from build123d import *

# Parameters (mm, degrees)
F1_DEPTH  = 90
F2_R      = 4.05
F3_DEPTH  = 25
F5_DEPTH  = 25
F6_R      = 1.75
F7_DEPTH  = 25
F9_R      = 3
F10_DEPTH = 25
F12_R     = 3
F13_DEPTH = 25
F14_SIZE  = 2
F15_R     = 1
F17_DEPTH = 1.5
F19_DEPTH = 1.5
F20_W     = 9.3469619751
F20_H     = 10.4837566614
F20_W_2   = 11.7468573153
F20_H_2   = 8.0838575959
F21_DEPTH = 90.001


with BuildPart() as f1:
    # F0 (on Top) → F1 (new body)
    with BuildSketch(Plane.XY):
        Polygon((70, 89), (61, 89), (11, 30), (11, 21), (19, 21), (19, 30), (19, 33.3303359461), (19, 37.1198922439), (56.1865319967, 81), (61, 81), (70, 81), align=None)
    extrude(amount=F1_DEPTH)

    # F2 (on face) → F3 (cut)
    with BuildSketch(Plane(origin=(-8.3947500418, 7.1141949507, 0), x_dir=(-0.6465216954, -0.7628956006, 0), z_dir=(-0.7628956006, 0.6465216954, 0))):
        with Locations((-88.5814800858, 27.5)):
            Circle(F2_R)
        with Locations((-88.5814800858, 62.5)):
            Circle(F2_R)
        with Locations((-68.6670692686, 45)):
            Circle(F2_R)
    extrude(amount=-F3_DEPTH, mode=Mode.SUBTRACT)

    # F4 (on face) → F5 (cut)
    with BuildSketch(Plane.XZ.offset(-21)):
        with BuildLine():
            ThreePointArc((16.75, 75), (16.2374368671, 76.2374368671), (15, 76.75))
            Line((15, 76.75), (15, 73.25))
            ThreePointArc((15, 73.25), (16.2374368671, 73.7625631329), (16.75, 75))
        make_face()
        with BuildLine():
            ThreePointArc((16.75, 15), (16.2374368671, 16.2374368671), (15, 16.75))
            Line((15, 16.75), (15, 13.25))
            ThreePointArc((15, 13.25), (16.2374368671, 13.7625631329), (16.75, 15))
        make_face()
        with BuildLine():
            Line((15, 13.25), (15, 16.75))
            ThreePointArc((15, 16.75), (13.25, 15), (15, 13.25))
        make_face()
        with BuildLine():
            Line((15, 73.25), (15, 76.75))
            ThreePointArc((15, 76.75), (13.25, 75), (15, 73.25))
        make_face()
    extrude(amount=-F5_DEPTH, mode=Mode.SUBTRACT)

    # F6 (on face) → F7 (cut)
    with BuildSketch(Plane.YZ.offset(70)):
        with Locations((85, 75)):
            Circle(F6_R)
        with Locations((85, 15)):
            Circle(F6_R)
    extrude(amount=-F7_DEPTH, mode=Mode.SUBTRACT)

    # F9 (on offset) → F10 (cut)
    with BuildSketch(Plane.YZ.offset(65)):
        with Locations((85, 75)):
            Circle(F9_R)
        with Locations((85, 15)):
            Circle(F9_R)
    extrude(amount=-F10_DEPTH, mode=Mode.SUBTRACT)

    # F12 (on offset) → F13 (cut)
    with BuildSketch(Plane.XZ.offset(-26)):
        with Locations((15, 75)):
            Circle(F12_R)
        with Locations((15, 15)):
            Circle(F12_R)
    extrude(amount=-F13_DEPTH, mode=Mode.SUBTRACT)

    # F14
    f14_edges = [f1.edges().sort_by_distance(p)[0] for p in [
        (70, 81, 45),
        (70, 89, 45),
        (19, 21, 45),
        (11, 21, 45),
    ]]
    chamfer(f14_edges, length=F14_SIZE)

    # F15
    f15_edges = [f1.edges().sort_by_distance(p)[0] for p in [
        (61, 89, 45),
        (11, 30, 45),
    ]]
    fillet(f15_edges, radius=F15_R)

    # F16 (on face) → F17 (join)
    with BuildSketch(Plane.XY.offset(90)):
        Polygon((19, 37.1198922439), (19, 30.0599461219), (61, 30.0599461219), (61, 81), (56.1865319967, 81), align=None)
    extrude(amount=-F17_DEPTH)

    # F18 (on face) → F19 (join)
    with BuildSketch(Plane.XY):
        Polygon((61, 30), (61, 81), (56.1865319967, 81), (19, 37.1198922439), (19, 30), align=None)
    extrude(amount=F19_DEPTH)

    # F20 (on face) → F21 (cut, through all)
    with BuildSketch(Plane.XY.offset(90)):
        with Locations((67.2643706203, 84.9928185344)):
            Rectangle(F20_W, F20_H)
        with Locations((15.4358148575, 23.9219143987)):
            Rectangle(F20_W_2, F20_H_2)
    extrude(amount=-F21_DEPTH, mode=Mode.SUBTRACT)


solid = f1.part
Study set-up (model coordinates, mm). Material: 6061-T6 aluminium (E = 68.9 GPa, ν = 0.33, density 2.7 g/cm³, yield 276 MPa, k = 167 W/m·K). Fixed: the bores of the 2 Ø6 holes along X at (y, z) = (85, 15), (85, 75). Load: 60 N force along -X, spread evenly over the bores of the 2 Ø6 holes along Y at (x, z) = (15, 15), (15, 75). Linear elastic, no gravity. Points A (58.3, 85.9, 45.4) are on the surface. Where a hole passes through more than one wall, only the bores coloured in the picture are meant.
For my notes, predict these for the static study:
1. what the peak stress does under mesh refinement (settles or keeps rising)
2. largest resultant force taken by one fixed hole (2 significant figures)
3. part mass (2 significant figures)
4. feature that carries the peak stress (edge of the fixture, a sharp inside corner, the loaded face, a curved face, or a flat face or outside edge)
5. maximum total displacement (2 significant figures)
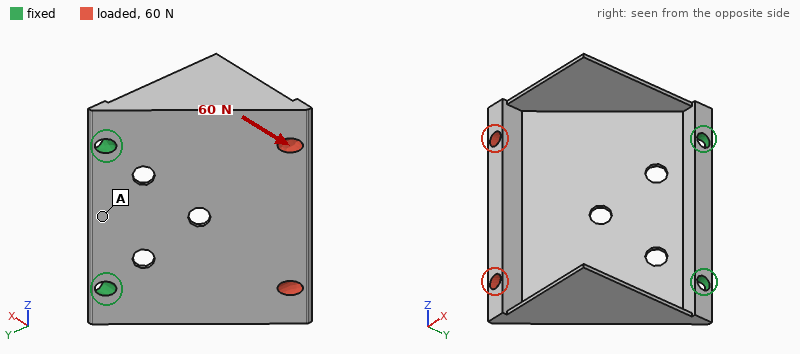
keeps rising
30 N
52 g
a sharp inside corner
0.36 mm
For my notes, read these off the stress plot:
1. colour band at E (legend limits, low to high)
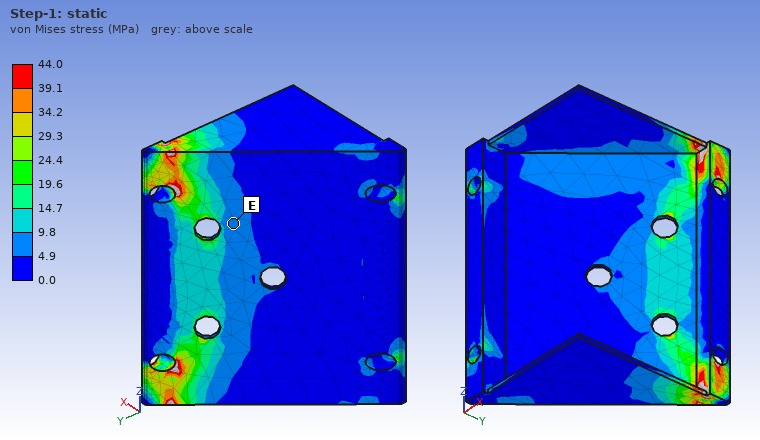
4.9 to 9.8 MPa
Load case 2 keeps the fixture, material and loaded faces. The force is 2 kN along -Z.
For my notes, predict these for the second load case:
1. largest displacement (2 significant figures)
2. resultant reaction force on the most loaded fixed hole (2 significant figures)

0.52 mm
2.3 kN
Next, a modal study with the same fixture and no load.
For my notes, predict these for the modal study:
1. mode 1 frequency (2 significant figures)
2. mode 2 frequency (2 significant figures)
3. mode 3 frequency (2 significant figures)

420 Hz
700 Hz
1300 Hz
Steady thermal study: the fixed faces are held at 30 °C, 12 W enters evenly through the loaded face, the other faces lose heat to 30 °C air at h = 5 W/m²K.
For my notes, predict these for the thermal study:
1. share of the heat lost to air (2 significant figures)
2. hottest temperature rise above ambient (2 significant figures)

13 %
30 K
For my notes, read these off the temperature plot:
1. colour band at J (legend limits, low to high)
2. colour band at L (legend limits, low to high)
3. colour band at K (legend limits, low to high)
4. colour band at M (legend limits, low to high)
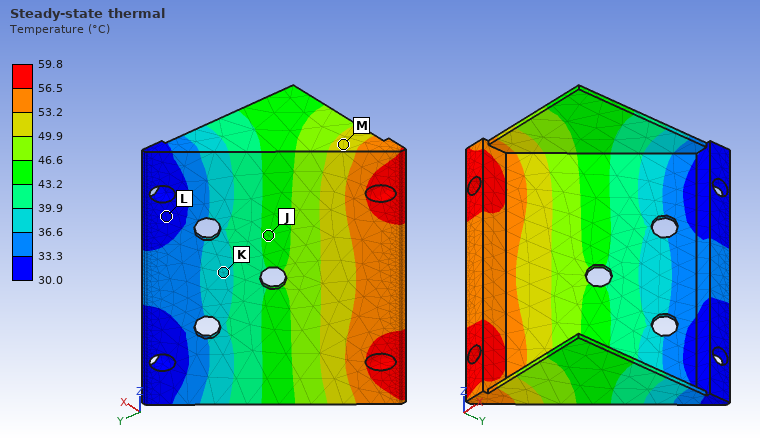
43.2 to 46.6 °C
30.0 to 33.3 °C
36.6 to 39.9 °C
49.9 to 53.2 °C
